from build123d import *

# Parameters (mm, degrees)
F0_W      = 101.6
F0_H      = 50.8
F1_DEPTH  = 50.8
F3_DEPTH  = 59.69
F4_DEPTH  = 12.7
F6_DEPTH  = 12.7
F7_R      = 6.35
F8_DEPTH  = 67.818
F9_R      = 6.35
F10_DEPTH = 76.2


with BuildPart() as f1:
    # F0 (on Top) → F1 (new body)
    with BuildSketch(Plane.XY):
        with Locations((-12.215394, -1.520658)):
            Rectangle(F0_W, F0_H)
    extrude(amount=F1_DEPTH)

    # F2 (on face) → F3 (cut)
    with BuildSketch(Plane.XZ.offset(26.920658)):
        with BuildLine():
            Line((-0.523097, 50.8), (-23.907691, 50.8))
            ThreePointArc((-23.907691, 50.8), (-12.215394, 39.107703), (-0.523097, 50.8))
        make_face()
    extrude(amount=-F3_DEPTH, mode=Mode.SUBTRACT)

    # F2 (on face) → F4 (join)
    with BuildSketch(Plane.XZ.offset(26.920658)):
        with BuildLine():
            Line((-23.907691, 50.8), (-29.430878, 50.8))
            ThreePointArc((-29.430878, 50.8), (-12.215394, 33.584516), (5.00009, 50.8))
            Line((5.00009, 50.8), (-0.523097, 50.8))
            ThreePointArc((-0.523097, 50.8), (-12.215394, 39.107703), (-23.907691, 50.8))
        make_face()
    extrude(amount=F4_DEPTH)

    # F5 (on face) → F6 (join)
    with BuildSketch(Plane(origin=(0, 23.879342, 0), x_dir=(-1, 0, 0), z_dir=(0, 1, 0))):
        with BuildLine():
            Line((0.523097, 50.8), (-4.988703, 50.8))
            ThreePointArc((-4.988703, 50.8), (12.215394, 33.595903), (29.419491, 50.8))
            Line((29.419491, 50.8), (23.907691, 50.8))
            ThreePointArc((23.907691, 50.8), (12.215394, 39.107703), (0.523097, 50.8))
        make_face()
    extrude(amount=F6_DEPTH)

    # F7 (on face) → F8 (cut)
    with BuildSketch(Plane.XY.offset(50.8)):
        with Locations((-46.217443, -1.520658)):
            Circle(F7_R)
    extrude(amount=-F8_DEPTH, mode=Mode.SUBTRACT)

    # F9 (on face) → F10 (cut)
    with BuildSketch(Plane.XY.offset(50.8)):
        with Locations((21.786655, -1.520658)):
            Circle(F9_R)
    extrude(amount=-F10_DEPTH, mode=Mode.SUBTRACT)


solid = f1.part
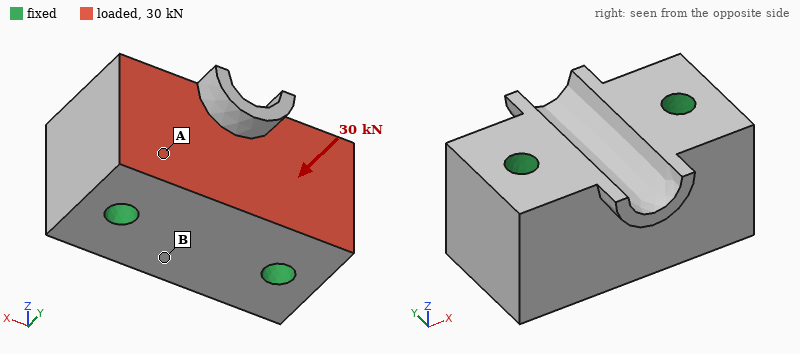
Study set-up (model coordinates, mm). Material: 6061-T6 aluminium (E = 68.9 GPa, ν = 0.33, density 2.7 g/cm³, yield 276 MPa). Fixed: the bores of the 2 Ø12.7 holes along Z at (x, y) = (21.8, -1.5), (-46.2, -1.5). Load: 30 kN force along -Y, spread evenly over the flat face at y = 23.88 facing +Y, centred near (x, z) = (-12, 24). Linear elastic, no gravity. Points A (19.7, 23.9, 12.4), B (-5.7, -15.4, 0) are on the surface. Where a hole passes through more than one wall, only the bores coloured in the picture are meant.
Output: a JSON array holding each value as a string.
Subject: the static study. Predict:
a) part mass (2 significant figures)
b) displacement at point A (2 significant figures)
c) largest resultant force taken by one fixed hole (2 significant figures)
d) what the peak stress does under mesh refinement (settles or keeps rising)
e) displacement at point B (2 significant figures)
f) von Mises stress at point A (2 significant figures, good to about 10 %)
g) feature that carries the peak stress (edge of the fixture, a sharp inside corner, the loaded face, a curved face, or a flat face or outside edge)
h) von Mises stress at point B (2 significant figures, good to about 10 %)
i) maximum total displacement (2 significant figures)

["660 g", "2.6 µm", "15 kN", "keeps rising", "3.2 µm", "8.7 MPa", "edge of the fixture", "2.8 MPa", "5.8 µm"]
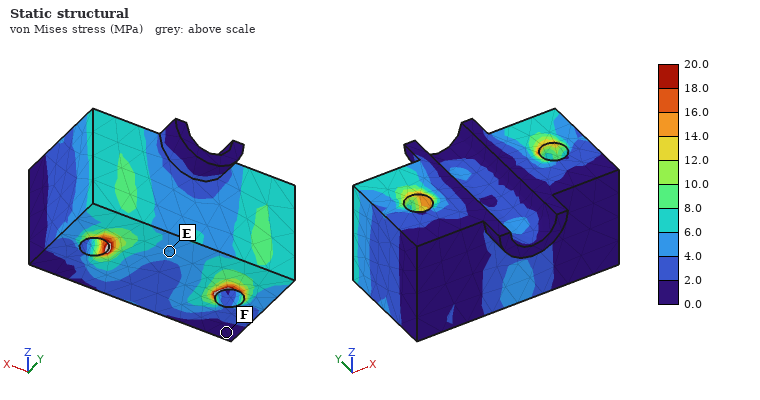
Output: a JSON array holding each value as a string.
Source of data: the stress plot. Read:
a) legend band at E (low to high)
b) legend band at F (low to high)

["4.0 to 6.0 MPa", "0.0 to 2.0 MPa"]
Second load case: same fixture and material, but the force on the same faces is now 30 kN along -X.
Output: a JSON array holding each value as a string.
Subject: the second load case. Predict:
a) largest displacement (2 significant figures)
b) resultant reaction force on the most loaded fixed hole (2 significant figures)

["13 µm", "17 kN"]
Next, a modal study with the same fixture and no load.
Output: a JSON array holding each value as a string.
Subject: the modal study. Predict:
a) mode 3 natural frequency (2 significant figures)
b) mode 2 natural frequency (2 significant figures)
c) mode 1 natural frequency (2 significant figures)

["18 kHz", "18 kHz", "18 kHz"]
